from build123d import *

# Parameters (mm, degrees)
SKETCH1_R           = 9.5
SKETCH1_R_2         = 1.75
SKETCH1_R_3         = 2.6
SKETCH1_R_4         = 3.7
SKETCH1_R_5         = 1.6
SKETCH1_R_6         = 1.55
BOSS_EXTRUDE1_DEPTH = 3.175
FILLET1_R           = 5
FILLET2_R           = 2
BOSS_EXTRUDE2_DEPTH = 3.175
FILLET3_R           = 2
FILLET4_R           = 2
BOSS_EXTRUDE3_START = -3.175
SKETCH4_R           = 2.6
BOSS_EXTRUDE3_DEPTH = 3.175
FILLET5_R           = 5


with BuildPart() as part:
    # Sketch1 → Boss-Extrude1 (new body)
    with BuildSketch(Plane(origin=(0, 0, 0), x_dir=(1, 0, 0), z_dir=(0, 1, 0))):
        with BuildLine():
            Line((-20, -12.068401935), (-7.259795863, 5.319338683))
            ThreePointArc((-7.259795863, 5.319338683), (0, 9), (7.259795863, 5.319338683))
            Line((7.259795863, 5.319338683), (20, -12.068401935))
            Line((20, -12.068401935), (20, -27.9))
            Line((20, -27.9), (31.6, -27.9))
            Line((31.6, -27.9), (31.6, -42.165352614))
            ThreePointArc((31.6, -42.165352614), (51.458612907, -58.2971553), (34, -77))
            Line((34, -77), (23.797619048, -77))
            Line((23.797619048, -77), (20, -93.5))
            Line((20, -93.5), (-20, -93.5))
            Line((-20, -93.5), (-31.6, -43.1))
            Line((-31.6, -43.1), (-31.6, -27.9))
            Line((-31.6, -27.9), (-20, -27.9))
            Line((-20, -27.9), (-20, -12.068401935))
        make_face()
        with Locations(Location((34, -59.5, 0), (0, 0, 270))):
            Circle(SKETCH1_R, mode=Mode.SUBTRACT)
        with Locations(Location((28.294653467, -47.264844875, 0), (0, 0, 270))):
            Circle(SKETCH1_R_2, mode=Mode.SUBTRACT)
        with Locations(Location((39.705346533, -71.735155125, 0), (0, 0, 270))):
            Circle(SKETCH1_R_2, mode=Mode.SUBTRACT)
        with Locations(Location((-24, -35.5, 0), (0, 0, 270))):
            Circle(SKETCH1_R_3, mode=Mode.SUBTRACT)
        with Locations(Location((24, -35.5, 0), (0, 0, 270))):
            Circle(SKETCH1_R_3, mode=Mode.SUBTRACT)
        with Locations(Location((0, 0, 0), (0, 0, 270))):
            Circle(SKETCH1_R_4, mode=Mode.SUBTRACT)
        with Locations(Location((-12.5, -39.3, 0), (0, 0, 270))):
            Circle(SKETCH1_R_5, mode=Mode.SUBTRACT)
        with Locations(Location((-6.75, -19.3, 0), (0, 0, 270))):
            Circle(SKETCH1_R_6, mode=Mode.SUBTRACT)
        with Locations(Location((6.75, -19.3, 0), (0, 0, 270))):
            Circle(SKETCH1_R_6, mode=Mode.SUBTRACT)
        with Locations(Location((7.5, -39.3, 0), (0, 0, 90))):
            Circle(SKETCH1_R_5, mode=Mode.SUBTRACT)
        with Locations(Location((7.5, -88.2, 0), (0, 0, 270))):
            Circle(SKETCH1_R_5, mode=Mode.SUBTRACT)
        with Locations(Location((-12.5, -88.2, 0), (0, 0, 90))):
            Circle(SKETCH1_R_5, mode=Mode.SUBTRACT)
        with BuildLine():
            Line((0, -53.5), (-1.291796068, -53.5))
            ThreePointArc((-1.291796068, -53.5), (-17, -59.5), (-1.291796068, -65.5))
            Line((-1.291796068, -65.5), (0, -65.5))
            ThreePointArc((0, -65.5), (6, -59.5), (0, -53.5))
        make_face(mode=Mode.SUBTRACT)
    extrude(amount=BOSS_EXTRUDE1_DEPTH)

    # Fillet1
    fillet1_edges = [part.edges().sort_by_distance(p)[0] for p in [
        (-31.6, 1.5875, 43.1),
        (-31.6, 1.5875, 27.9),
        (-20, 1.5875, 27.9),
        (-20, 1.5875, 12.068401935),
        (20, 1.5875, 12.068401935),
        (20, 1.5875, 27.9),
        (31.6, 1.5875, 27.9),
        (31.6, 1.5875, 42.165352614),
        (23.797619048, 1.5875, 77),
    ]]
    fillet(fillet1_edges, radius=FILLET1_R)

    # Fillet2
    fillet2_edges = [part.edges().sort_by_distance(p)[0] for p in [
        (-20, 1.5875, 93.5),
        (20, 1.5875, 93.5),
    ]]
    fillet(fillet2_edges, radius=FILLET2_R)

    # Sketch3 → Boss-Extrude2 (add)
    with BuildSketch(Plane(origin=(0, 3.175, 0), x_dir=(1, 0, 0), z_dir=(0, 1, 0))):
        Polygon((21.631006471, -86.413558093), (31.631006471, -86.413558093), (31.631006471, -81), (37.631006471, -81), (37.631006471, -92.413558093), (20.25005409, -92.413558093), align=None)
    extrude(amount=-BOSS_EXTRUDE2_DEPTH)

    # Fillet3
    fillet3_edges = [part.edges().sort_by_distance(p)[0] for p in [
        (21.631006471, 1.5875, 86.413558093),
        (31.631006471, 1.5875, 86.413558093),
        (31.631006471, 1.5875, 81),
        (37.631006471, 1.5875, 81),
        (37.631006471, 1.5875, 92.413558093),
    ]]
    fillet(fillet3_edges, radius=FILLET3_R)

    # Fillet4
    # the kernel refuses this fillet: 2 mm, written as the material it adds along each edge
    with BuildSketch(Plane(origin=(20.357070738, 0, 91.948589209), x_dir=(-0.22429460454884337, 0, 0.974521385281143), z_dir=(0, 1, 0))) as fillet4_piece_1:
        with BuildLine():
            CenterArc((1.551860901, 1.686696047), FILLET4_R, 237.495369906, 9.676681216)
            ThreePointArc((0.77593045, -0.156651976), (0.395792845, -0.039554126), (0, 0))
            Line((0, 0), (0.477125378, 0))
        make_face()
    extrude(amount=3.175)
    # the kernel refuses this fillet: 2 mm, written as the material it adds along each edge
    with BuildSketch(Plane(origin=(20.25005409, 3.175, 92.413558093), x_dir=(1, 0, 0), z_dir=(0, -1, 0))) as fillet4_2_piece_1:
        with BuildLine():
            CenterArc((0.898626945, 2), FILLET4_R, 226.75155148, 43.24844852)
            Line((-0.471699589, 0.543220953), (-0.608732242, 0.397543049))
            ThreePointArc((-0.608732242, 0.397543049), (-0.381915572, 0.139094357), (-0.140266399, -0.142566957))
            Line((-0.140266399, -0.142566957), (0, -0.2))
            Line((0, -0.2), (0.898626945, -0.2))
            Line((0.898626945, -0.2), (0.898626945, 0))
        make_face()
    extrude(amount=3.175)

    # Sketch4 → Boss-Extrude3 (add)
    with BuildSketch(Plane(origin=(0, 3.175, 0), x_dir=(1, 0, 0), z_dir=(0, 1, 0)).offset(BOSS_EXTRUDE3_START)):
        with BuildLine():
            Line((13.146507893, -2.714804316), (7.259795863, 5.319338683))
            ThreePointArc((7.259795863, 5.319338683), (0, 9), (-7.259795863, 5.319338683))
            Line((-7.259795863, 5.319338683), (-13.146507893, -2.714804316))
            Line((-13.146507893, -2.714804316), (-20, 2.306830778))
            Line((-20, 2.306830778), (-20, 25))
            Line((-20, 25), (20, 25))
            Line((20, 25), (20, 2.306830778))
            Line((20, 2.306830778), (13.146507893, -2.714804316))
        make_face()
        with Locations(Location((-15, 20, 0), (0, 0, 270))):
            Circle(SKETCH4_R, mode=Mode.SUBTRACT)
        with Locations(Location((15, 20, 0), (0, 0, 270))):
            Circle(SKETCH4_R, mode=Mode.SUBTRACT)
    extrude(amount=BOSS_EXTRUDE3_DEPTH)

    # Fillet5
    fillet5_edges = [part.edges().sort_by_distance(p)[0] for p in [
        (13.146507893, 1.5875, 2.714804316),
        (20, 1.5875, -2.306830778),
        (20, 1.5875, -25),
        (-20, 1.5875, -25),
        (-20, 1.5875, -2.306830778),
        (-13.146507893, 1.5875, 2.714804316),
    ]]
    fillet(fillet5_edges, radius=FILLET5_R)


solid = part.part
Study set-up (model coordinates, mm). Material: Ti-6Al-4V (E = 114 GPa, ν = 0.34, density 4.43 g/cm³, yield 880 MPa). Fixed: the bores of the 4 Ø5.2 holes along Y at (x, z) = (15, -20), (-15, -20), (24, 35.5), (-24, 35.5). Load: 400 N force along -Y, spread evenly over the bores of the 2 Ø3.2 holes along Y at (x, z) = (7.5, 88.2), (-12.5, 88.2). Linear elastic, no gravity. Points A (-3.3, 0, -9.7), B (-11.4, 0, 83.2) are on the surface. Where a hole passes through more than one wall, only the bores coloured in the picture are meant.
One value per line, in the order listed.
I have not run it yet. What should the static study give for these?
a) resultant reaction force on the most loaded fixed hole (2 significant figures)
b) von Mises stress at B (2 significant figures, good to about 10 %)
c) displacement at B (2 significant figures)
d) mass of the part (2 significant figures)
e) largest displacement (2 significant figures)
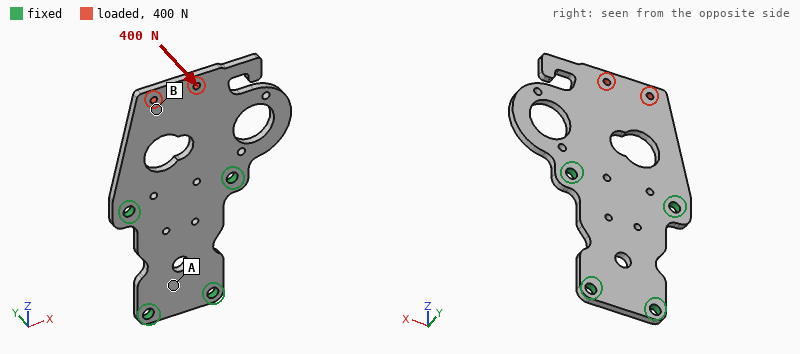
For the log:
250 N
61 MPa
1.2 mm
79 g
1.6 mm
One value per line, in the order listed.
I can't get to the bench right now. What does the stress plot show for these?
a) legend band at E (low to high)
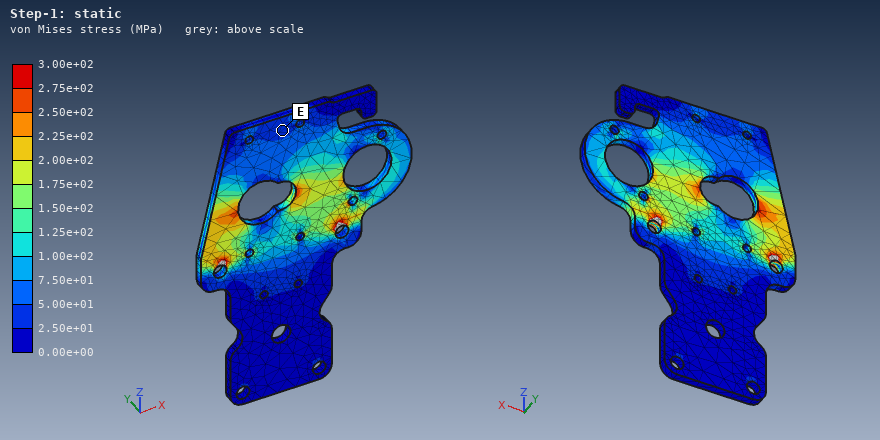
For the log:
2.50e+01 to 5.00e+01 MPa
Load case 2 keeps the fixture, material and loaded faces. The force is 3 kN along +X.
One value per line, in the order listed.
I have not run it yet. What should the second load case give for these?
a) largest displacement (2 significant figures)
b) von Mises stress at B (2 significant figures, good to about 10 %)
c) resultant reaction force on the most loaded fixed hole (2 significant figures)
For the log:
78 µm
59 MPa
3.5 kN
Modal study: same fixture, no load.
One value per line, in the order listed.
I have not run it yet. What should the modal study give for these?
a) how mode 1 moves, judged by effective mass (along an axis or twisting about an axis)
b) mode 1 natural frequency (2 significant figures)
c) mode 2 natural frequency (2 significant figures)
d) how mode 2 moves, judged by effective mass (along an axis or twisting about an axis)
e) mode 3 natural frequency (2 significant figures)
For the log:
along Y
740 Hz
1700 Hz
twisting about Z
2900 Hz
